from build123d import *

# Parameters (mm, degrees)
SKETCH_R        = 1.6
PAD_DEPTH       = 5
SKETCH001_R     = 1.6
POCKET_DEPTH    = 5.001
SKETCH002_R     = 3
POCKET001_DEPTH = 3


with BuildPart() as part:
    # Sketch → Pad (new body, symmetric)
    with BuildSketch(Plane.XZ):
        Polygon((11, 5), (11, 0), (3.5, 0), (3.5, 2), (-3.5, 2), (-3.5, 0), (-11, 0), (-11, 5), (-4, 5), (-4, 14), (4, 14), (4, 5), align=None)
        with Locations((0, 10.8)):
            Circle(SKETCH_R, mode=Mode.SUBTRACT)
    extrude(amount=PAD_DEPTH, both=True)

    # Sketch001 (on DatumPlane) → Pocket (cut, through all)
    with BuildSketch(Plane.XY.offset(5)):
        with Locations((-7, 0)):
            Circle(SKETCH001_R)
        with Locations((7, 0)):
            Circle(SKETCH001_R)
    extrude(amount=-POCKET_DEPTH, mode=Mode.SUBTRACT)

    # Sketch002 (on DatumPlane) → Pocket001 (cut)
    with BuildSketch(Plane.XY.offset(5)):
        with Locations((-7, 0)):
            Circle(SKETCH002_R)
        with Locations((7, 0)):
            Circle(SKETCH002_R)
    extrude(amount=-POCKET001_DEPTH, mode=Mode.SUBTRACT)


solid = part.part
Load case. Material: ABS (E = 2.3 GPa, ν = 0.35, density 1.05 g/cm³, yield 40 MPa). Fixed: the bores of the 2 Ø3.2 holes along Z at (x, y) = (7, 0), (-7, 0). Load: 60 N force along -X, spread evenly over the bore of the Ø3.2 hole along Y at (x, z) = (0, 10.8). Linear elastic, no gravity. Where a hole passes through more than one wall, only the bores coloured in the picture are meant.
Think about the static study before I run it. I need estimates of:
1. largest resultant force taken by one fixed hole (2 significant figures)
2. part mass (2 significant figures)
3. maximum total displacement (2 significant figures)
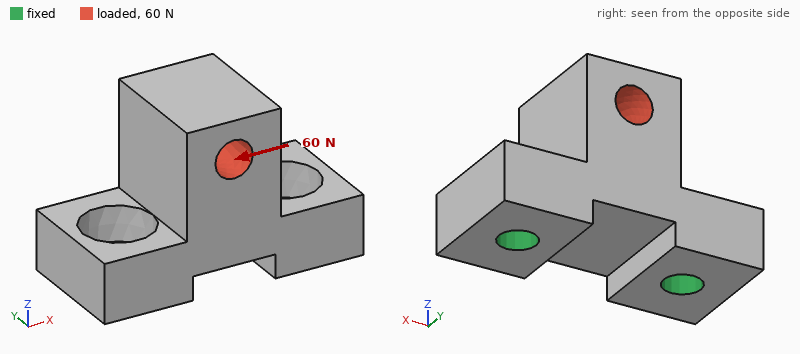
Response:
57 N
1.5 g
58 µm
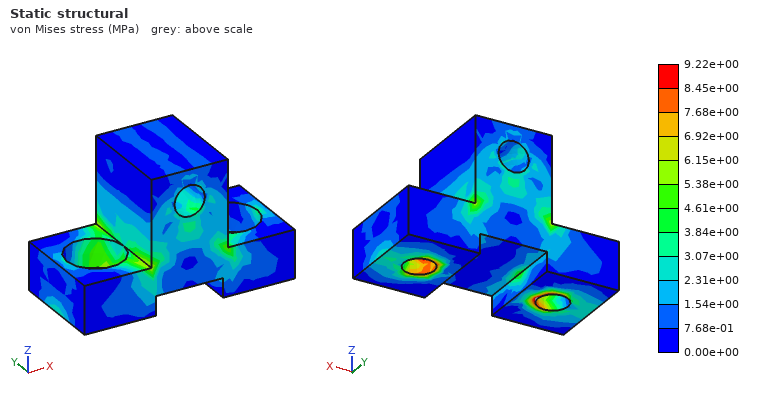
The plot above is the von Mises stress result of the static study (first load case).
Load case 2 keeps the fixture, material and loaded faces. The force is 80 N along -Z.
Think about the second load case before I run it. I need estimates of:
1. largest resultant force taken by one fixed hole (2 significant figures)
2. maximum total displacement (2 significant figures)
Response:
47 N
19 µm
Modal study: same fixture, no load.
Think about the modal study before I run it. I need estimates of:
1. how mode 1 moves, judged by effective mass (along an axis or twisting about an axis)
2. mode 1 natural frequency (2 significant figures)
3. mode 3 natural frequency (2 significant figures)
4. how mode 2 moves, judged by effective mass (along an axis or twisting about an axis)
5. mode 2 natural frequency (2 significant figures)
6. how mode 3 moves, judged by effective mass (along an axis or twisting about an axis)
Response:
along Y
3900 Hz
12 kHz
along X
8100 Hz
along Z
